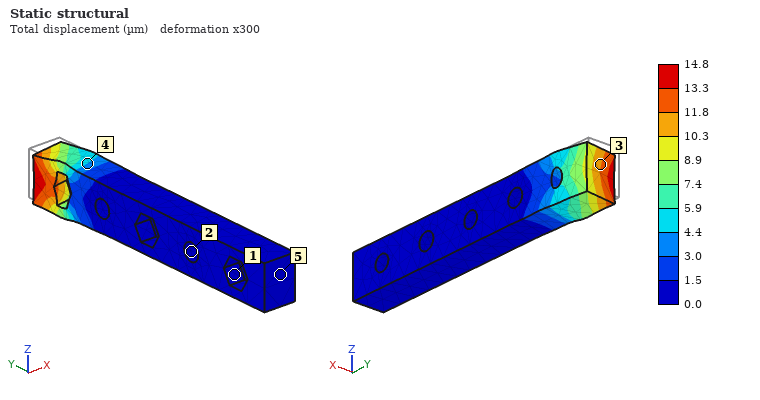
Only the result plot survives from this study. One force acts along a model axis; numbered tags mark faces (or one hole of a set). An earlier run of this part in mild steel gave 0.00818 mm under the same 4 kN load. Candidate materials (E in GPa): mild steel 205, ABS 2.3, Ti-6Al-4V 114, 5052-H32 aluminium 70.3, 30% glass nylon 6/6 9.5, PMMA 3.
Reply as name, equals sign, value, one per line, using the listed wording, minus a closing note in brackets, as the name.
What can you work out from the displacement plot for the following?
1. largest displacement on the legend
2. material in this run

largest displacement on the legend = 14.8 µm
material in this run = Ti-6Al-4V
